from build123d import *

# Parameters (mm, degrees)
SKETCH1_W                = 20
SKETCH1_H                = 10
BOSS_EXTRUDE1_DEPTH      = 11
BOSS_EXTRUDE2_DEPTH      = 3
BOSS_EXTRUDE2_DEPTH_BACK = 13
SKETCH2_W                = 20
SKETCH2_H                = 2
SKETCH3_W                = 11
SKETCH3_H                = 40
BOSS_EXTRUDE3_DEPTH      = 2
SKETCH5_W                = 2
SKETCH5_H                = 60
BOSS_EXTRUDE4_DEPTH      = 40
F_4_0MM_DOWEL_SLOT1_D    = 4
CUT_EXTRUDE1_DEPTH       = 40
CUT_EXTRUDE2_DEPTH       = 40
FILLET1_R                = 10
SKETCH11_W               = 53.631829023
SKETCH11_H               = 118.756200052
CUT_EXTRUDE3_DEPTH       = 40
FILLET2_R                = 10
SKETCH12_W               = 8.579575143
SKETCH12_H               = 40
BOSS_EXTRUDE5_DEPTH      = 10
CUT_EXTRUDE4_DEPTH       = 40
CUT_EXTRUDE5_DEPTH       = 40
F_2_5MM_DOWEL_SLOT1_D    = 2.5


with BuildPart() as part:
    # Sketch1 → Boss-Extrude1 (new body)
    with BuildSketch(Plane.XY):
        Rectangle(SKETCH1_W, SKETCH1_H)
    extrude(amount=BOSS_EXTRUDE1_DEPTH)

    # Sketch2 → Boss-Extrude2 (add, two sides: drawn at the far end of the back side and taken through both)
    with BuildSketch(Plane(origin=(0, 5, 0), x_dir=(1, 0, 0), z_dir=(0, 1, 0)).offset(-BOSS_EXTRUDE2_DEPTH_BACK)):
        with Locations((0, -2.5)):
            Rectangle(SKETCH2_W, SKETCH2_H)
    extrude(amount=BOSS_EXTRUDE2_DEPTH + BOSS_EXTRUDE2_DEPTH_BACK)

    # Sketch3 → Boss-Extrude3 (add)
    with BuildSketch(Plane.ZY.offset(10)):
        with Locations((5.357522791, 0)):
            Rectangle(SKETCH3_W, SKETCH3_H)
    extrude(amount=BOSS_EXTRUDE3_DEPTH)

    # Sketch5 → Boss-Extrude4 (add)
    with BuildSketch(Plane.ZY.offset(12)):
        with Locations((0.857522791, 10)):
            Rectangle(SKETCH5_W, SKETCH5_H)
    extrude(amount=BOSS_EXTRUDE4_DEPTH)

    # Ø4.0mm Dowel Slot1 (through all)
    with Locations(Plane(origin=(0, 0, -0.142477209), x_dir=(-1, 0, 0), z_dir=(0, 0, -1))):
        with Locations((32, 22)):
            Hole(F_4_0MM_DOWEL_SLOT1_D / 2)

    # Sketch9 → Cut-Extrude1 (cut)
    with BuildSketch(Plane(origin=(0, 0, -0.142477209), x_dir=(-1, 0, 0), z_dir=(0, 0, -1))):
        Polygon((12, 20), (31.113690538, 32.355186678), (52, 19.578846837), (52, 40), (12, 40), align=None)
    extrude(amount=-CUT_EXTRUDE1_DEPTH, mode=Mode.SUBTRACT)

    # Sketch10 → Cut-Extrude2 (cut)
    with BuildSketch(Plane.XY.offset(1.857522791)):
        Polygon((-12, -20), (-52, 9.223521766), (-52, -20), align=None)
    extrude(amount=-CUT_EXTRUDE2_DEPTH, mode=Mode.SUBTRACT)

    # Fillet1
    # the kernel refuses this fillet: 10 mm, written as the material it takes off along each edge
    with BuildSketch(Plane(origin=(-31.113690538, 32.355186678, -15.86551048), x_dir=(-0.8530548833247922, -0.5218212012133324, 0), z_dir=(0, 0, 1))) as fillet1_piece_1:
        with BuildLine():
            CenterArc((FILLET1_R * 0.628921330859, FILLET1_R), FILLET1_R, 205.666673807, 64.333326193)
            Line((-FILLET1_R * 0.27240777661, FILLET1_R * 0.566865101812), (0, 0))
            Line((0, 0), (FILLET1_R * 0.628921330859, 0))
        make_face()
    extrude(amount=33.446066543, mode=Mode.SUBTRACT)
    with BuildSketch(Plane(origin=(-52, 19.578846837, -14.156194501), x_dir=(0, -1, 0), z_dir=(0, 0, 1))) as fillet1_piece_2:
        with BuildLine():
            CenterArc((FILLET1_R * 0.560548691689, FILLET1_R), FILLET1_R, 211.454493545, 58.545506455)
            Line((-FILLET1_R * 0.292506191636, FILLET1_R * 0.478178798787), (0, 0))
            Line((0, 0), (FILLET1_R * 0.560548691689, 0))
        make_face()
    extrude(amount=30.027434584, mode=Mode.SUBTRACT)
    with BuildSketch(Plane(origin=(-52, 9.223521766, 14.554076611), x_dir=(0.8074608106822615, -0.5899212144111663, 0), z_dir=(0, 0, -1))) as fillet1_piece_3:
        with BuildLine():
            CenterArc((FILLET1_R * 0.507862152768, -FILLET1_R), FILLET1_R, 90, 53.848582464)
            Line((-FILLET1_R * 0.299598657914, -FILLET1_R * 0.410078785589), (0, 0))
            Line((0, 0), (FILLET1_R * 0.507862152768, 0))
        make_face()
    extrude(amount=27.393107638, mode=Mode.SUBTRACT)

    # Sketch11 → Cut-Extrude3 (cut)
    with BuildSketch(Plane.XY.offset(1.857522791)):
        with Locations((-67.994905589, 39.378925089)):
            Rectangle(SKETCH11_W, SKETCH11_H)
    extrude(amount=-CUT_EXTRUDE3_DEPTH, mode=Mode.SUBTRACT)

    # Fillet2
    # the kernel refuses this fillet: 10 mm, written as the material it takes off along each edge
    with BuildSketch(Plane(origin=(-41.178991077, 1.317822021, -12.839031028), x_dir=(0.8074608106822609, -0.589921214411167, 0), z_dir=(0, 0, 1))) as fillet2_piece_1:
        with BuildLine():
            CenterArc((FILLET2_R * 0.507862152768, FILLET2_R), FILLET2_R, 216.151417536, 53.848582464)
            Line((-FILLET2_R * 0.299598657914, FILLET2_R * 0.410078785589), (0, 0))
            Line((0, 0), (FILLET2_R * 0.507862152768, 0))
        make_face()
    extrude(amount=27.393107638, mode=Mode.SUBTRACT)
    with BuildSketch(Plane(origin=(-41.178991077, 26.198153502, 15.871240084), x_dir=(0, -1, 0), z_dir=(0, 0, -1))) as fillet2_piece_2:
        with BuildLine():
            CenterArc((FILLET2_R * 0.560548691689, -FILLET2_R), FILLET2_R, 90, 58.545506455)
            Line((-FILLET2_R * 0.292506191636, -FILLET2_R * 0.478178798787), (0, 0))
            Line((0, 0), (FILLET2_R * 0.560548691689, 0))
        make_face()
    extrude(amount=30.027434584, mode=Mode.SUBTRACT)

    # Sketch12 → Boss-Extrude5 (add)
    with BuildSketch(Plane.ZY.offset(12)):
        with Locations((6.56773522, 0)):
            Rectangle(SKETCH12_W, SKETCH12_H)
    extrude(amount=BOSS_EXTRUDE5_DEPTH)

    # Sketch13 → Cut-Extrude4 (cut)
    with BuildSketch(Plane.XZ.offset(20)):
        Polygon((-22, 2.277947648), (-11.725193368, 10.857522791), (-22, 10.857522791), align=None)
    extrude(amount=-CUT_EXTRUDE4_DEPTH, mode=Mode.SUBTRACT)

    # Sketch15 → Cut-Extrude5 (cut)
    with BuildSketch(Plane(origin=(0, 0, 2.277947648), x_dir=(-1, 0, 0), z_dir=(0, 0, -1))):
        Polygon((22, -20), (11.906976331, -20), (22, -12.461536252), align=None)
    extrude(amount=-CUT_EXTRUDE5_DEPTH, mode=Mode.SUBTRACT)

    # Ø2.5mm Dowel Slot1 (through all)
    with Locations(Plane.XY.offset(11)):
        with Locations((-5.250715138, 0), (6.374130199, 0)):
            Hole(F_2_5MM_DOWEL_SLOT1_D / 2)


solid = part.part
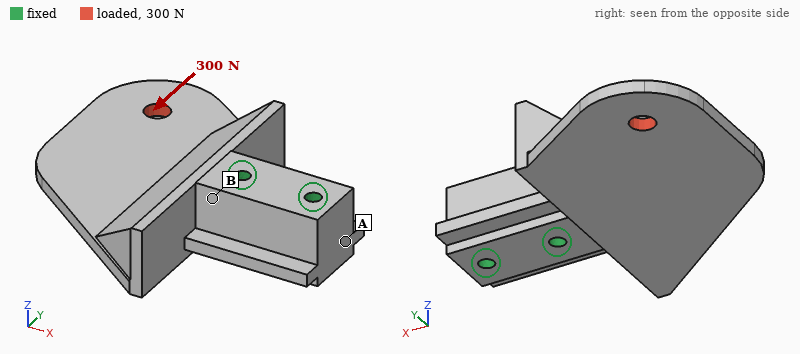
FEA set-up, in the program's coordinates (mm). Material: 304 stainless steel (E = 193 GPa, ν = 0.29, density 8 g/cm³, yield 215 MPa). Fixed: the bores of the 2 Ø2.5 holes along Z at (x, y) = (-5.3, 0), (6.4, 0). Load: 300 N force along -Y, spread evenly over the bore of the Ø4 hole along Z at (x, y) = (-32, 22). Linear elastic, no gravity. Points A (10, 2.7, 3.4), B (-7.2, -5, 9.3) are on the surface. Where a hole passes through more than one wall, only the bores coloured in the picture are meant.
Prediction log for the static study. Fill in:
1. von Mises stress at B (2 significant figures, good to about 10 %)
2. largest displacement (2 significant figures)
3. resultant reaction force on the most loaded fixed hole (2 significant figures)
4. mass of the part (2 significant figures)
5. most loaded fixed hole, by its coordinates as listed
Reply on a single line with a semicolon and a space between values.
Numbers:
23 MPa; 23 µm; 770 N; 55 g; (-5.3, 0)
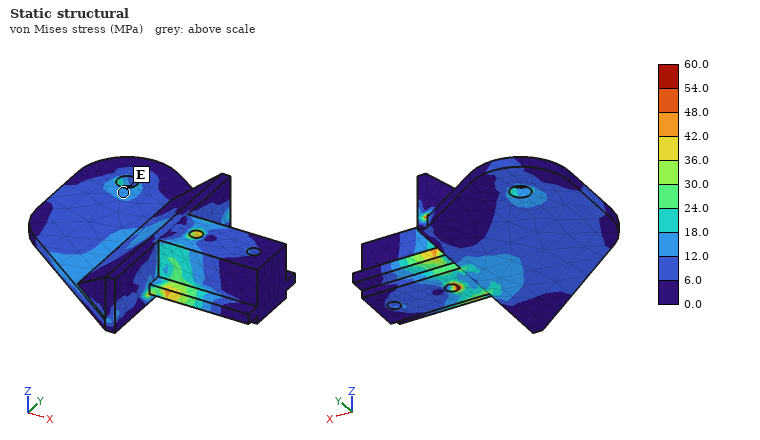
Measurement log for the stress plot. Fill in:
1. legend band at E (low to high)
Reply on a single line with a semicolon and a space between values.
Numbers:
12.0 to 18.0 MPa
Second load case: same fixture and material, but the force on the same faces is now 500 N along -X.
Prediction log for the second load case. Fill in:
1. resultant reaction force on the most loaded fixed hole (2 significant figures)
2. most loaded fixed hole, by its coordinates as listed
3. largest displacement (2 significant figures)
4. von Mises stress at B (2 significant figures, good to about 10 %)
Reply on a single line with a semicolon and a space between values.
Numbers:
780 N; (-5.3, 0); 40 µm; 33 MPa
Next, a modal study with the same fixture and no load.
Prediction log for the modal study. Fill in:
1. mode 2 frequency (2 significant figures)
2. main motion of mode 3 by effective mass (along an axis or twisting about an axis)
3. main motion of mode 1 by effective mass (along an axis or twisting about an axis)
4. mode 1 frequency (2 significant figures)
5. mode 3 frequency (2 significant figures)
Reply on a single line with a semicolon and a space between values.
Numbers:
4000 Hz; along Y; along Z; 1600 Hz; 5500 Hz
